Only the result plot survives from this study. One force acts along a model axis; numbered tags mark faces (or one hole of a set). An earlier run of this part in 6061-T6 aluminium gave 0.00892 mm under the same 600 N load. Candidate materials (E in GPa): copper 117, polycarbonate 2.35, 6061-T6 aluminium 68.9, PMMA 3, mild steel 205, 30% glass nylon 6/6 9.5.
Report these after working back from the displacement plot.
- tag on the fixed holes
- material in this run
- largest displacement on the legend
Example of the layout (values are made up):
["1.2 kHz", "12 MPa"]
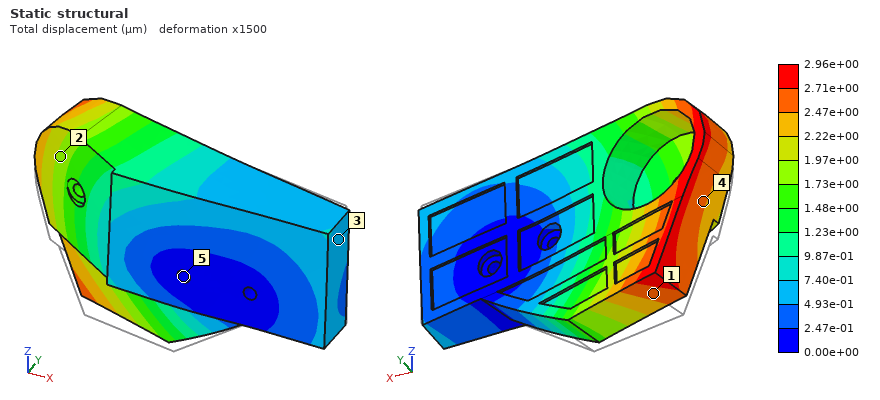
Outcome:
["5", "mild steel", "2.96e+00 µm"]
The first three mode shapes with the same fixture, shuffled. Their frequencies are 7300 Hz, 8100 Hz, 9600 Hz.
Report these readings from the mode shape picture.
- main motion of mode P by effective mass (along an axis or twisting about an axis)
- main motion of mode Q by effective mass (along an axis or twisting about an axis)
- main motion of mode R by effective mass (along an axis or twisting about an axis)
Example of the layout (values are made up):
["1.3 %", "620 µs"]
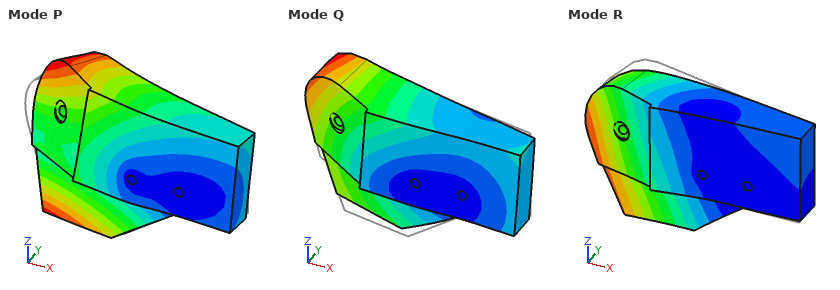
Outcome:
["twisting about X", "along Z", "along Y"]
